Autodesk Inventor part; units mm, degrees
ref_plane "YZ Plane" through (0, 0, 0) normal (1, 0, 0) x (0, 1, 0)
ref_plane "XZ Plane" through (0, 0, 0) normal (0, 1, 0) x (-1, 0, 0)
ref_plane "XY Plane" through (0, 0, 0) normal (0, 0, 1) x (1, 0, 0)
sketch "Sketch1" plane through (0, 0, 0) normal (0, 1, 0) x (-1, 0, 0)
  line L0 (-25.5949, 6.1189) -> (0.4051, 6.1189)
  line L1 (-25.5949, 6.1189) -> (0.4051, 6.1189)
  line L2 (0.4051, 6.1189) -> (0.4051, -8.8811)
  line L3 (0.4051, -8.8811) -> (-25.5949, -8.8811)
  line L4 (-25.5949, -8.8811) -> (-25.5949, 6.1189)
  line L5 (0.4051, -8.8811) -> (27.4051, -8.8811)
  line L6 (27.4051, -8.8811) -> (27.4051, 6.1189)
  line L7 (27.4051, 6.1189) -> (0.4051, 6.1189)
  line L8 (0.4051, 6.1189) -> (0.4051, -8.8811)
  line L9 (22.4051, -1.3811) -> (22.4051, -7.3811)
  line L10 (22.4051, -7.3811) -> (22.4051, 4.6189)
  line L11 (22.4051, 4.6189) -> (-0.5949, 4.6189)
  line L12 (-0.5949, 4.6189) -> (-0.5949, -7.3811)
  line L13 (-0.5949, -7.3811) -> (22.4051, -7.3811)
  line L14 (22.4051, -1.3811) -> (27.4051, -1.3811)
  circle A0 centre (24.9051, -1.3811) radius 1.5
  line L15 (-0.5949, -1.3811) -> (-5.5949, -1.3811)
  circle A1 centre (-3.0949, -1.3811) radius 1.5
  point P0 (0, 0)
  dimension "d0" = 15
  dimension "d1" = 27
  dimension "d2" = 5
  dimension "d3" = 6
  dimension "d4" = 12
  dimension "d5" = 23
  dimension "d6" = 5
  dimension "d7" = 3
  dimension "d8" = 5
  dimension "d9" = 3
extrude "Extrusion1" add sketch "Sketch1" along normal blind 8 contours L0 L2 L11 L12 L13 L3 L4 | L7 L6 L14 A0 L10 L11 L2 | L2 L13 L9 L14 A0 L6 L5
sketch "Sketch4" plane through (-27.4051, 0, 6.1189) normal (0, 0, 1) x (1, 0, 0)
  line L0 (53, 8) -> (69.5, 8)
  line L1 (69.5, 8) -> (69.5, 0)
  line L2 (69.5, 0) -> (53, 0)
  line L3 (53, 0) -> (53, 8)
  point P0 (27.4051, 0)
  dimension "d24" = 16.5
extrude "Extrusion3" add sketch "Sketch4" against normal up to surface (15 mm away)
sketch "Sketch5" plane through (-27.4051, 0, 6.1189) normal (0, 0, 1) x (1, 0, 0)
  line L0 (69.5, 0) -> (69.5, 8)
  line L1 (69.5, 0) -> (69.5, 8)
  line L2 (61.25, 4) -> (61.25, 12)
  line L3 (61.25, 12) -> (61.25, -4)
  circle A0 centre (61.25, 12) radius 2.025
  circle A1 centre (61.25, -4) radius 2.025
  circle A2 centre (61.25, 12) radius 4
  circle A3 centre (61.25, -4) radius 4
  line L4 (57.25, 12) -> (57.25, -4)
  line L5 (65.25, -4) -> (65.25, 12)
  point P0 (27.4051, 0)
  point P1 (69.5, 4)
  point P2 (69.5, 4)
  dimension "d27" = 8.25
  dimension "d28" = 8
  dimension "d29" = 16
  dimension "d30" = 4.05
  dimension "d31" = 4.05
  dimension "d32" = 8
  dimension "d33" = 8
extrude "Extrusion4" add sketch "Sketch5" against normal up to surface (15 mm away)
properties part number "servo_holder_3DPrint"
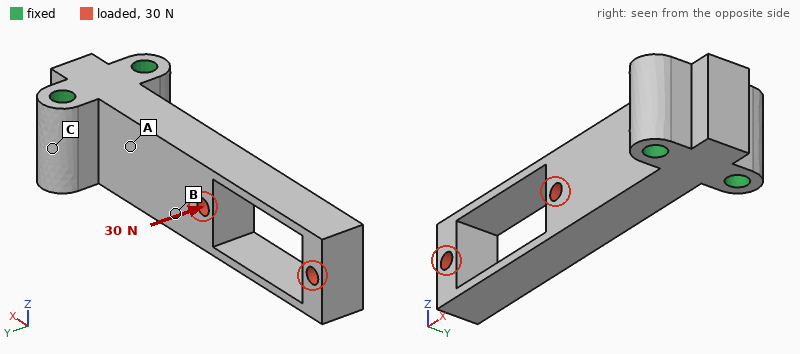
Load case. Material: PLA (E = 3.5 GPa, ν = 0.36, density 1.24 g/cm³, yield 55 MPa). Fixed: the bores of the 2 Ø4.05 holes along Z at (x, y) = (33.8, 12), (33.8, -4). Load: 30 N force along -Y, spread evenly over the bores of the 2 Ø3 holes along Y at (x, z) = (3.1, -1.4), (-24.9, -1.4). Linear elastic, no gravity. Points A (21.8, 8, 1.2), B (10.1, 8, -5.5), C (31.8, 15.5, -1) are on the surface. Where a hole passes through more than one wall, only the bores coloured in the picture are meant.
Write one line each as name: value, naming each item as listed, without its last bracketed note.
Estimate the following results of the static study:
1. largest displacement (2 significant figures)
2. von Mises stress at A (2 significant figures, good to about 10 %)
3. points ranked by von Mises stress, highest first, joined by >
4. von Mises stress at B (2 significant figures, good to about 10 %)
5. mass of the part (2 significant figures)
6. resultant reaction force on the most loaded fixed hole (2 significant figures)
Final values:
largest displacement: 0.83 mm
von Mises stress at A: 6.1 MPa
points ranked by von Mises stress, highest first, joined by >: A > B > C
von Mises stress at B: 4.0 MPa
mass of the part: 9.1 g
resultant reaction force on the most loaded fixed hole: 100 N
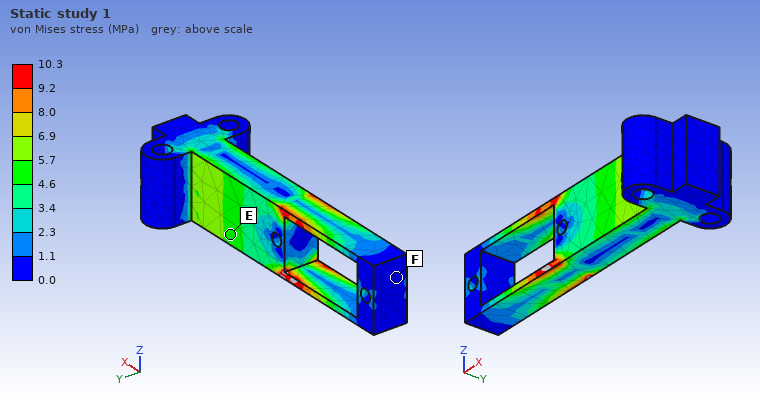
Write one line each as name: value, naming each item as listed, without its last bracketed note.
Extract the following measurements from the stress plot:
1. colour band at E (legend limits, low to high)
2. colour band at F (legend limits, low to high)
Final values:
colour band at E: 4.6 to 5.7 MPa
colour band at F: 0.0 to 1.1 MPa
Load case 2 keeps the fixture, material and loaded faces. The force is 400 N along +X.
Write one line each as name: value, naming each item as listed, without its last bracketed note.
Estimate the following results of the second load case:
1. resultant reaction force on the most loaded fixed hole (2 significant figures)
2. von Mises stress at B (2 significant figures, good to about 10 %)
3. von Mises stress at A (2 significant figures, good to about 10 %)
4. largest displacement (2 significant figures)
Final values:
resultant reaction force on the most loaded fixed hole: 210 N
von Mises stress at B: 3.3 MPa
von Mises stress at A: 3.3 MPa
largest displacement: 0.15 mm
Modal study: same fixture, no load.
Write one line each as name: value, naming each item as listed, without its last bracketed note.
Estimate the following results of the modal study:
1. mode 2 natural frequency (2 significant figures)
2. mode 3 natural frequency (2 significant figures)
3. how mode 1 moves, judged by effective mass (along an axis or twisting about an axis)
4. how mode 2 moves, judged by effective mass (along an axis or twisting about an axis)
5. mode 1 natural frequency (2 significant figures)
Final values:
mode 2 natural frequency: 780 Hz
mode 3 natural frequency: 2300 Hz
how mode 1 moves, judged by effective mass: along Z
how mode 2 moves, judged by effective mass: along Y
mode 1 natural frequency: 560 Hz
